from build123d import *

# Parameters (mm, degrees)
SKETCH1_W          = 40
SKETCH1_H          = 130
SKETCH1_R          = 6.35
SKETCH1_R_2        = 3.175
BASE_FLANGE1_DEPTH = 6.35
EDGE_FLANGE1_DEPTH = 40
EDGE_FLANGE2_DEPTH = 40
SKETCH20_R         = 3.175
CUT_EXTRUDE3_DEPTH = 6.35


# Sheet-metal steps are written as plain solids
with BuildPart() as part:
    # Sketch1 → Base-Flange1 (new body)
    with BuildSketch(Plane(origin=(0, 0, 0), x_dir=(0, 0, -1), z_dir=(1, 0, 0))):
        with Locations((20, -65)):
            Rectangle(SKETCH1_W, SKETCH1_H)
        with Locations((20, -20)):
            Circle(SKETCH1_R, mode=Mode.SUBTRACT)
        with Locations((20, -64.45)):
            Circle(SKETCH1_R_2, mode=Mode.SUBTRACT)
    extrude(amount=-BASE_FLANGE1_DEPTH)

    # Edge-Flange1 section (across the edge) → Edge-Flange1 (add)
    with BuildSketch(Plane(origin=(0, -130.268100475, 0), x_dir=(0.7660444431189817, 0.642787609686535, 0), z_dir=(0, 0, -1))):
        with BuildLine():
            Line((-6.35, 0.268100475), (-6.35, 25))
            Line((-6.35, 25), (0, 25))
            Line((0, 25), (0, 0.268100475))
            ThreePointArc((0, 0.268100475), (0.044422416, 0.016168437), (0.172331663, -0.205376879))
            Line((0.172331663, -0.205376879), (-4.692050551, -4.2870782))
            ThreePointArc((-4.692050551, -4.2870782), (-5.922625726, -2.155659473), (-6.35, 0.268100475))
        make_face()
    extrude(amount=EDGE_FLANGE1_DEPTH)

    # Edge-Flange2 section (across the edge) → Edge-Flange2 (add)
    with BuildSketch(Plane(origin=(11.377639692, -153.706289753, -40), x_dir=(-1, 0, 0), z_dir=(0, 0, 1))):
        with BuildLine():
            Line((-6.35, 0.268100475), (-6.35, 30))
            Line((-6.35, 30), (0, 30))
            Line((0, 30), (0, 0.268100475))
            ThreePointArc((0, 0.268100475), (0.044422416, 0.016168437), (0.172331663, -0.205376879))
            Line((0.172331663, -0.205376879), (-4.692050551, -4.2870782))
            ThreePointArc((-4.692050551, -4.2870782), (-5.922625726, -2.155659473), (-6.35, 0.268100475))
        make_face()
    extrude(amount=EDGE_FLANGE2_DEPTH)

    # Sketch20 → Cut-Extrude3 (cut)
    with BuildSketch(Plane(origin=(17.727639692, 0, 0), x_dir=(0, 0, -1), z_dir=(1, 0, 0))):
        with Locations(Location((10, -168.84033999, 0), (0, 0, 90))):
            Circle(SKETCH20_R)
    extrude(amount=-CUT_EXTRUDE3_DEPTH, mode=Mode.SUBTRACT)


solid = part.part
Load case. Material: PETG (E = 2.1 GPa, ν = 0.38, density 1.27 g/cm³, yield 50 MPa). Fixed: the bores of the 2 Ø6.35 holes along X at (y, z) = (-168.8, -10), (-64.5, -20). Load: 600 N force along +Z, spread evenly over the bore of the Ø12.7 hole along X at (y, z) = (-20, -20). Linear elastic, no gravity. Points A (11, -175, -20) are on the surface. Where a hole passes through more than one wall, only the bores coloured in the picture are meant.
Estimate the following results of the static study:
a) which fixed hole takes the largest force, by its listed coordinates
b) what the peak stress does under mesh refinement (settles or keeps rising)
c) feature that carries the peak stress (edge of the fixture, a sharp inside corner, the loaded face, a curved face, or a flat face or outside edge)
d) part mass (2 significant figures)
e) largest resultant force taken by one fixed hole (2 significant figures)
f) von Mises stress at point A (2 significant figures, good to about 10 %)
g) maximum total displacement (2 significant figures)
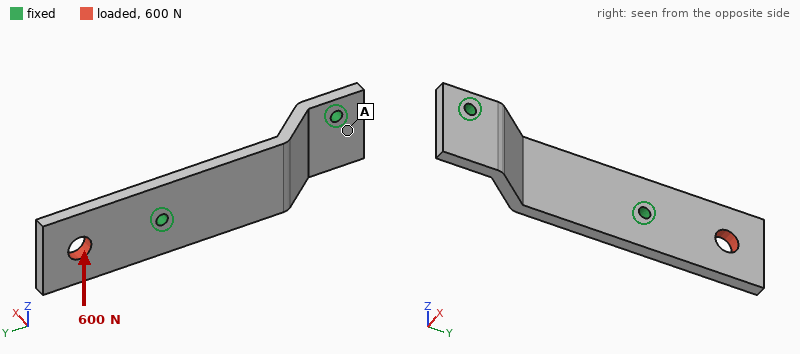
(-64.5, -20)
keeps rising
edge of the fixture
60 g
790 N
4.1 MPa
1.7 mm
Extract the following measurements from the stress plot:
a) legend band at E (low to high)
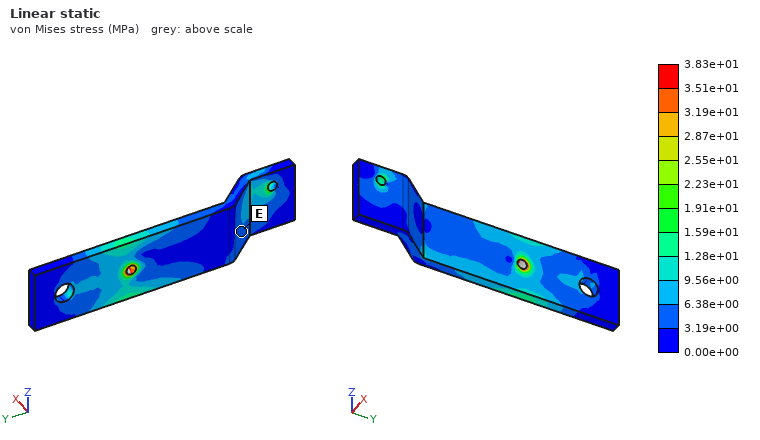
3.19e+00 to 6.38e+00 MPa
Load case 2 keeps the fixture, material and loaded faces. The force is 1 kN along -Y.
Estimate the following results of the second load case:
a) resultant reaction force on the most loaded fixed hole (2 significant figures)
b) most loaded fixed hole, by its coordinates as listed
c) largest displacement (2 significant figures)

980 N
(-64.5, -20)
0.15 mm
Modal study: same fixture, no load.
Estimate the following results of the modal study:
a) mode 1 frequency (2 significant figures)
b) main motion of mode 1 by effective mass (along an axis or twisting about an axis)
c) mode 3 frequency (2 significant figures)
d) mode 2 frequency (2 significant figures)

320 Hz
along X
890 Hz
710 Hz
